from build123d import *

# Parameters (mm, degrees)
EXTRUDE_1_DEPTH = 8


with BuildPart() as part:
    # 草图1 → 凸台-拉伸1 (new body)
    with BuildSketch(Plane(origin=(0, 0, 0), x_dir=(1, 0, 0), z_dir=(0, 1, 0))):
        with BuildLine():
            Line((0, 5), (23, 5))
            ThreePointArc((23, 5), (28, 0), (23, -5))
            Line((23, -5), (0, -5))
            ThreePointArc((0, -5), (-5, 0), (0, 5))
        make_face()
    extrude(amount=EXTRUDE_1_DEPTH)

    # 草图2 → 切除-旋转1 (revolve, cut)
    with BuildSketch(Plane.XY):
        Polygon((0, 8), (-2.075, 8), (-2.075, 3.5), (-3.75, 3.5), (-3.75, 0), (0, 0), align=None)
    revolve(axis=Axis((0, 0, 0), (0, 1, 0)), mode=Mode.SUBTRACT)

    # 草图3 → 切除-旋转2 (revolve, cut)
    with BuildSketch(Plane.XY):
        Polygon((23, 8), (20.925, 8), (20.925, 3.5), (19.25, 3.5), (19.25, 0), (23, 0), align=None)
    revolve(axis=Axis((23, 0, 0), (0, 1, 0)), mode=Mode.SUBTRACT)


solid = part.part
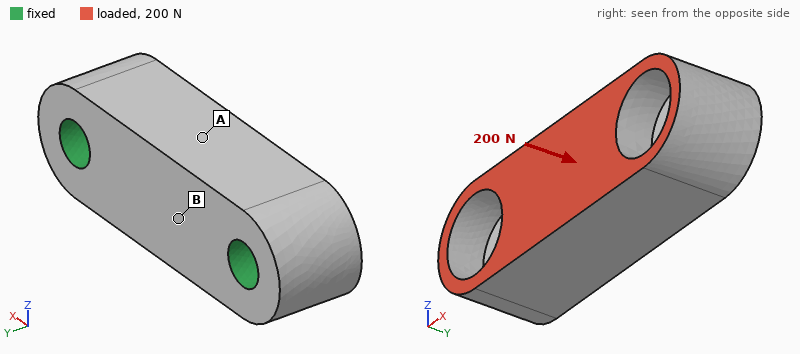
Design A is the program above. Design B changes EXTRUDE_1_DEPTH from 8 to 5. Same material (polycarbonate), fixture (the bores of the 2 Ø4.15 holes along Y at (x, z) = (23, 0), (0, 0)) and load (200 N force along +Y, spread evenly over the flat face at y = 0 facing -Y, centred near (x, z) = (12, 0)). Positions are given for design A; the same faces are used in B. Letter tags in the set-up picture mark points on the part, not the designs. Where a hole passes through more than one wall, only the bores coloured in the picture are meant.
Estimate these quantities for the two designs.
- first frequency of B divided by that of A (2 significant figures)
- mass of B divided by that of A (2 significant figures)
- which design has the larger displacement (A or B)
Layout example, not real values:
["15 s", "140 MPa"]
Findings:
["0.65", "0.59", "B"]
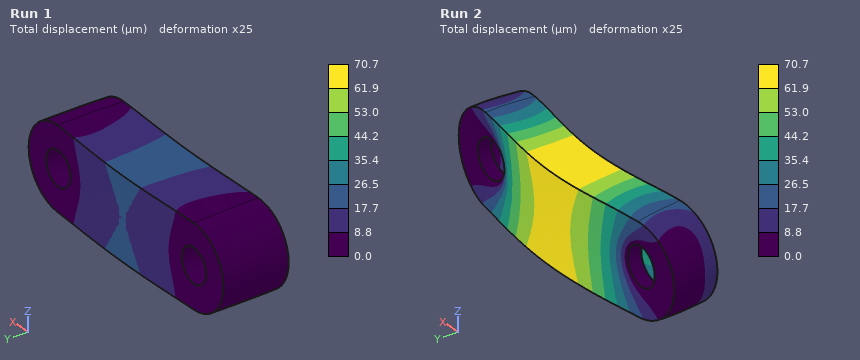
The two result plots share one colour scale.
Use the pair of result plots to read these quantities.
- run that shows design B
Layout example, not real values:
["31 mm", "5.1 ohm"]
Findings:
["Run 2"]
